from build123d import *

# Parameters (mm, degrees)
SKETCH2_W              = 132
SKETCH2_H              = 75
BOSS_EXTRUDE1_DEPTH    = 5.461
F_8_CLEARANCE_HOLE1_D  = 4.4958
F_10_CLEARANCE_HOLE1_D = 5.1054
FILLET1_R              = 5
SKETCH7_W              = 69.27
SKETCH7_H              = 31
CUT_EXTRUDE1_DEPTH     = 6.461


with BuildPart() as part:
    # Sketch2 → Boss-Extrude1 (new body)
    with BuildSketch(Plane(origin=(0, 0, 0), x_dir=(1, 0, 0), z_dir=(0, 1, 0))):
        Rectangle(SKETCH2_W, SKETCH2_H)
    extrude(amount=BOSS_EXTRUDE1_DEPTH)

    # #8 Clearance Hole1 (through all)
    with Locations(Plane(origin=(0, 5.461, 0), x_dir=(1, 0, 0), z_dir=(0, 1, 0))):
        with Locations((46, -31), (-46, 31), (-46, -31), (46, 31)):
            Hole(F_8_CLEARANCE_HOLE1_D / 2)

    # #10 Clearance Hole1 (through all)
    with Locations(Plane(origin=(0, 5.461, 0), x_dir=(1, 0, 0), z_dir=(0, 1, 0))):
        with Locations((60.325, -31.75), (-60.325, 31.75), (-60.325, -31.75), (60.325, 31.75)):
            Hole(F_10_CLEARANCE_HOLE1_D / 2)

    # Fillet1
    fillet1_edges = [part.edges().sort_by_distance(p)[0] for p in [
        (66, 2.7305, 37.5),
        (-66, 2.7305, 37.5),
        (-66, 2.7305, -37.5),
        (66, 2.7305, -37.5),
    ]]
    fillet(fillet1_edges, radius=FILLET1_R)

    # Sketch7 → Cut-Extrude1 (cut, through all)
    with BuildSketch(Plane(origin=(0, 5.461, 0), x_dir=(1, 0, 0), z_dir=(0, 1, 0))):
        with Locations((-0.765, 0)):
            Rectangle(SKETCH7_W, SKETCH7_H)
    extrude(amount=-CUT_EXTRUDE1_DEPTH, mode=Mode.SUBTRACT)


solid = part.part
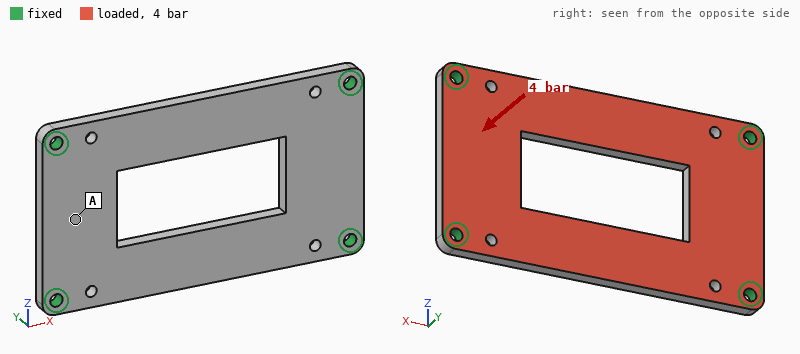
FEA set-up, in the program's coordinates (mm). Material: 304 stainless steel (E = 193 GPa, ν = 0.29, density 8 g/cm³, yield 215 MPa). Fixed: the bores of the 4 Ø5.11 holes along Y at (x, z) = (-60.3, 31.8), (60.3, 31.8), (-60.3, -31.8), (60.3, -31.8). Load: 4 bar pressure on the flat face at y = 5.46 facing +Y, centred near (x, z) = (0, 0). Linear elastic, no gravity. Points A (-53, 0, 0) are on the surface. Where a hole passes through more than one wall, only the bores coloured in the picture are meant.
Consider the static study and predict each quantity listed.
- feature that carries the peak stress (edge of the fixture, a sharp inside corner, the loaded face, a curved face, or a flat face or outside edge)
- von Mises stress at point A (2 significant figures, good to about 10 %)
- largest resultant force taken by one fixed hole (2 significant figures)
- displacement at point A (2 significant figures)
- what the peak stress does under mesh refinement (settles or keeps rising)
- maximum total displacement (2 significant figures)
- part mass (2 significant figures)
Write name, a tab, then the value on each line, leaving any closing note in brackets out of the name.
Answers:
feature that carries the peak stress	edge of the fixture
von Mises stress at point A	24 MPa
largest resultant force taken by one fixed hole	760 N
displacement at point A	0.022 mm
what the peak stress does under mesh refinement	keeps rising
maximum total displacement	0.11 mm
part mass	330 g
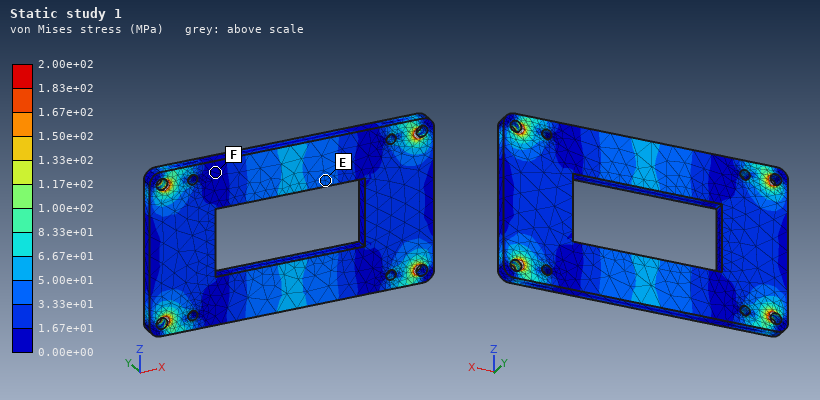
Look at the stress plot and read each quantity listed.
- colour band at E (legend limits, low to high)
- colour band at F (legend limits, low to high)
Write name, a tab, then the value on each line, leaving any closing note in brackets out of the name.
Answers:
colour band at E	3.33e+01 to 5.00e+01 MPa
colour band at F	0.00e+00 to 1.67e+01 MPa
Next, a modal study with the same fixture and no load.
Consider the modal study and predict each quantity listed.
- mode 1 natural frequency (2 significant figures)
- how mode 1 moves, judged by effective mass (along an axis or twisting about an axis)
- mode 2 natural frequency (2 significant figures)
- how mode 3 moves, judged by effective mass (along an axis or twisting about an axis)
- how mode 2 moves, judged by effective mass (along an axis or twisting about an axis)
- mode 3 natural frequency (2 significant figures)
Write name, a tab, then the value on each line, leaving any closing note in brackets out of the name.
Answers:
mode 1 natural frequency	1800 Hz
how mode 1 moves, judged by effective mass	along Y
mode 2 natural frequency	2300 Hz
how mode 3 moves, judged by effective mass	twisting about Z
how mode 2 moves, judged by effective mass	twisting about X
mode 3 natural frequency	4300 Hz
